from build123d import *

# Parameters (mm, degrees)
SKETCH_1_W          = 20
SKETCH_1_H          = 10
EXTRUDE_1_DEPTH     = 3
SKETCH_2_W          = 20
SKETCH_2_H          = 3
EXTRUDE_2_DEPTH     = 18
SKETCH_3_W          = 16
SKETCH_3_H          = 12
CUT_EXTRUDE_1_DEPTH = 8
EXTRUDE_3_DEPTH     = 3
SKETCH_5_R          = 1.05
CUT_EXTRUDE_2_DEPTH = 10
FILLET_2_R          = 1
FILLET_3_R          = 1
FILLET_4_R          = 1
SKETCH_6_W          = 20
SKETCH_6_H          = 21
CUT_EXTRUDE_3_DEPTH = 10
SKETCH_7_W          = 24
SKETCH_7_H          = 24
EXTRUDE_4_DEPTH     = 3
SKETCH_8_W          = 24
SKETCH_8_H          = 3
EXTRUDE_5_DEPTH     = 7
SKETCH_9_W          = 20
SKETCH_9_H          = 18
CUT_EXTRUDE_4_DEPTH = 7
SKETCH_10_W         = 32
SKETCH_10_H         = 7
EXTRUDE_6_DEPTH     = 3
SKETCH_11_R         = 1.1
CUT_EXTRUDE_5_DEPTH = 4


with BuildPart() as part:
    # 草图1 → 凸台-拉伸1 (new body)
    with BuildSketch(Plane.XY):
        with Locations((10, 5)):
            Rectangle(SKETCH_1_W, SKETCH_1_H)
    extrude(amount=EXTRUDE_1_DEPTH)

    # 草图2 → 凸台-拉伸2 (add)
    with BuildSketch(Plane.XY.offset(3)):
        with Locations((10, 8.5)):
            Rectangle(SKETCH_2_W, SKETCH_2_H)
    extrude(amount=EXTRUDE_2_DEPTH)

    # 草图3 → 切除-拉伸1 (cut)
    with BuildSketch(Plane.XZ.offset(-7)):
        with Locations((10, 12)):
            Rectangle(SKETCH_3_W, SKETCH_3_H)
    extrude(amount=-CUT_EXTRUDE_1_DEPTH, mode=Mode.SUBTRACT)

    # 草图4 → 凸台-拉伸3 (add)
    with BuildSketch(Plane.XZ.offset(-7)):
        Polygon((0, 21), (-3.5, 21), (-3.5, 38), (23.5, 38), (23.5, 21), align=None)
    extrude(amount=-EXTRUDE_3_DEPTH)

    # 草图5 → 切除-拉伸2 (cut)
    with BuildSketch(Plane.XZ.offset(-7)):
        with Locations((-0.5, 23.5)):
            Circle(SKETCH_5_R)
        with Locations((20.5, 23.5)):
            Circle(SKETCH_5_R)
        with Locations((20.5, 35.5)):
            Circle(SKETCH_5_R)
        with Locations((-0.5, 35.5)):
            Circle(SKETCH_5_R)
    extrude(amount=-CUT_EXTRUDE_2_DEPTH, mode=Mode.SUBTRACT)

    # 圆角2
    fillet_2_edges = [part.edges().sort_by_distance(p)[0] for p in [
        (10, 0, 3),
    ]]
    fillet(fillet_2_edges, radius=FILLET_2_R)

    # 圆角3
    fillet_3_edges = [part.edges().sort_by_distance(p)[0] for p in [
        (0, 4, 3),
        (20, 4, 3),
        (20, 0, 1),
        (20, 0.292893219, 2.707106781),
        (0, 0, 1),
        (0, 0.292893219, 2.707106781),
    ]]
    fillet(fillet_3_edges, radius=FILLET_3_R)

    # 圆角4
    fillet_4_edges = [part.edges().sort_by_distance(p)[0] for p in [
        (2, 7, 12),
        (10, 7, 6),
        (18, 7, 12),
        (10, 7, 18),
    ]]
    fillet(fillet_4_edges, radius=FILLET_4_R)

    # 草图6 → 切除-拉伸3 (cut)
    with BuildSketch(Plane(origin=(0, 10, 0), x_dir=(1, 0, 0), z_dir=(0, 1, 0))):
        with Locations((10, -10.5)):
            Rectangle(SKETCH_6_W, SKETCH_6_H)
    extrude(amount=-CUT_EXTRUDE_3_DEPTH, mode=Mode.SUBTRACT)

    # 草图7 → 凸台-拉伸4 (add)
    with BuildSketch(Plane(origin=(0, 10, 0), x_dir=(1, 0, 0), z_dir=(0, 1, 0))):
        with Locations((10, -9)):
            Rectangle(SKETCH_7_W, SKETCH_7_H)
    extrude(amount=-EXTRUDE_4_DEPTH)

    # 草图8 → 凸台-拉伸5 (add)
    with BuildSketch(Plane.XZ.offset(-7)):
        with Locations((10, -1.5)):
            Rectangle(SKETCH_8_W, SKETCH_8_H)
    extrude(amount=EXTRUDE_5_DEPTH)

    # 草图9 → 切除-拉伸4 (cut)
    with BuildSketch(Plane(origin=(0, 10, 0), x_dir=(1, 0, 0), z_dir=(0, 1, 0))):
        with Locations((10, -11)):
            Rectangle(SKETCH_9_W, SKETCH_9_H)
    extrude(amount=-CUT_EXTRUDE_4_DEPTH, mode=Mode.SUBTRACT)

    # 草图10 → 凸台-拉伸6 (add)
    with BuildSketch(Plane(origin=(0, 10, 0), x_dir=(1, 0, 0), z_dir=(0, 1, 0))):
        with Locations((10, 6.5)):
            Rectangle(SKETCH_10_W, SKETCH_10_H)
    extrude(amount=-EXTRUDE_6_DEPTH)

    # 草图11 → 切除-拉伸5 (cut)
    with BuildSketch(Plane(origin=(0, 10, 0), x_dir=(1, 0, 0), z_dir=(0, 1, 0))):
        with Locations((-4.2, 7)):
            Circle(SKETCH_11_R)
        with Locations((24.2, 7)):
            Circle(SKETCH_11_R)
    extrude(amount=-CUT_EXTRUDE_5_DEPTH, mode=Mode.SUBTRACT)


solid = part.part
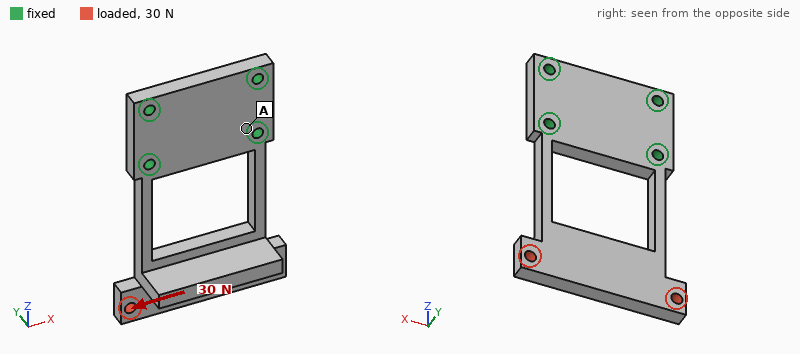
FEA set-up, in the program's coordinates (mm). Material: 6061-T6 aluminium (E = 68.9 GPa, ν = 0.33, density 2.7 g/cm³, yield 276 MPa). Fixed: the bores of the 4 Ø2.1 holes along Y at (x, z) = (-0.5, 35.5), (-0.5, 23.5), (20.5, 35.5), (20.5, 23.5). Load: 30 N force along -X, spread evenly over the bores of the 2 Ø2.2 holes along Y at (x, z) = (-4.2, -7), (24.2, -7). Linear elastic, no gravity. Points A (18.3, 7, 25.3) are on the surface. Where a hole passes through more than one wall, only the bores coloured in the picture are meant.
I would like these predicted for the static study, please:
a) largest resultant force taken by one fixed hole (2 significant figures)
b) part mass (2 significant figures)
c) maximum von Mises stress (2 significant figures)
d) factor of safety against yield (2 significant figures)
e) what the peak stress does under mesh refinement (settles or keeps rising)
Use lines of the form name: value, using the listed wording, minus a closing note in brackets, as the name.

largest resultant force taken by one fixed hole: 38 N
part mass: 8.5 g
maximum von Mises stress: 64 MPa
factor of safety against yield: 4.3
what the peak stress does under mesh refinement: settles
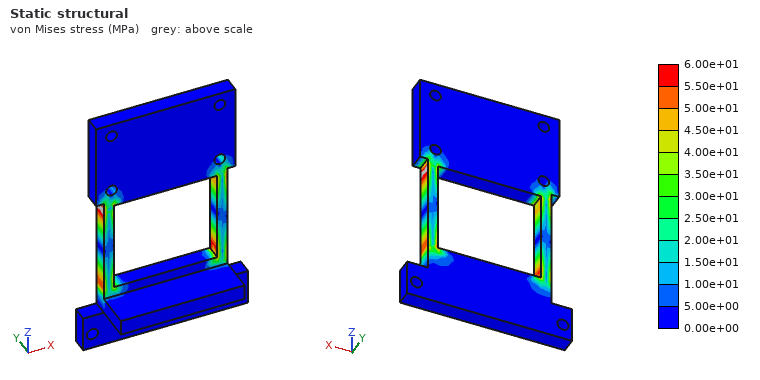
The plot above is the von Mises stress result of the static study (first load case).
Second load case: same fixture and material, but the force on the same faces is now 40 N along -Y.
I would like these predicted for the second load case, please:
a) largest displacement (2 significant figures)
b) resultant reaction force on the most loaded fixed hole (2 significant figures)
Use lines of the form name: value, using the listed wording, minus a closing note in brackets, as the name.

largest displacement: 0.59 mm
resultant reaction force on the most loaded fixed hole: 27 N
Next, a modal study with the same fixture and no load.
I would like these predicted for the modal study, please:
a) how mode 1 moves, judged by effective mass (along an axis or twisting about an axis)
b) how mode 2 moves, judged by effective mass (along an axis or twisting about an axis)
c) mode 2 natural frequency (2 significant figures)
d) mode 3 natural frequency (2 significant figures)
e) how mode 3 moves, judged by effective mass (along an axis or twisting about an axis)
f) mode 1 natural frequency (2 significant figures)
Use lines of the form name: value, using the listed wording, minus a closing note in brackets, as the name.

how mode 1 moves, judged by effective mass: along Y
how mode 2 moves, judged by effective mass: along X
mode 2 natural frequency: 1500 Hz
mode 3 natural frequency: 2600 Hz
how mode 3 moves, judged by effective mass: twisting about Z
mode 1 natural frequency: 810 Hz
